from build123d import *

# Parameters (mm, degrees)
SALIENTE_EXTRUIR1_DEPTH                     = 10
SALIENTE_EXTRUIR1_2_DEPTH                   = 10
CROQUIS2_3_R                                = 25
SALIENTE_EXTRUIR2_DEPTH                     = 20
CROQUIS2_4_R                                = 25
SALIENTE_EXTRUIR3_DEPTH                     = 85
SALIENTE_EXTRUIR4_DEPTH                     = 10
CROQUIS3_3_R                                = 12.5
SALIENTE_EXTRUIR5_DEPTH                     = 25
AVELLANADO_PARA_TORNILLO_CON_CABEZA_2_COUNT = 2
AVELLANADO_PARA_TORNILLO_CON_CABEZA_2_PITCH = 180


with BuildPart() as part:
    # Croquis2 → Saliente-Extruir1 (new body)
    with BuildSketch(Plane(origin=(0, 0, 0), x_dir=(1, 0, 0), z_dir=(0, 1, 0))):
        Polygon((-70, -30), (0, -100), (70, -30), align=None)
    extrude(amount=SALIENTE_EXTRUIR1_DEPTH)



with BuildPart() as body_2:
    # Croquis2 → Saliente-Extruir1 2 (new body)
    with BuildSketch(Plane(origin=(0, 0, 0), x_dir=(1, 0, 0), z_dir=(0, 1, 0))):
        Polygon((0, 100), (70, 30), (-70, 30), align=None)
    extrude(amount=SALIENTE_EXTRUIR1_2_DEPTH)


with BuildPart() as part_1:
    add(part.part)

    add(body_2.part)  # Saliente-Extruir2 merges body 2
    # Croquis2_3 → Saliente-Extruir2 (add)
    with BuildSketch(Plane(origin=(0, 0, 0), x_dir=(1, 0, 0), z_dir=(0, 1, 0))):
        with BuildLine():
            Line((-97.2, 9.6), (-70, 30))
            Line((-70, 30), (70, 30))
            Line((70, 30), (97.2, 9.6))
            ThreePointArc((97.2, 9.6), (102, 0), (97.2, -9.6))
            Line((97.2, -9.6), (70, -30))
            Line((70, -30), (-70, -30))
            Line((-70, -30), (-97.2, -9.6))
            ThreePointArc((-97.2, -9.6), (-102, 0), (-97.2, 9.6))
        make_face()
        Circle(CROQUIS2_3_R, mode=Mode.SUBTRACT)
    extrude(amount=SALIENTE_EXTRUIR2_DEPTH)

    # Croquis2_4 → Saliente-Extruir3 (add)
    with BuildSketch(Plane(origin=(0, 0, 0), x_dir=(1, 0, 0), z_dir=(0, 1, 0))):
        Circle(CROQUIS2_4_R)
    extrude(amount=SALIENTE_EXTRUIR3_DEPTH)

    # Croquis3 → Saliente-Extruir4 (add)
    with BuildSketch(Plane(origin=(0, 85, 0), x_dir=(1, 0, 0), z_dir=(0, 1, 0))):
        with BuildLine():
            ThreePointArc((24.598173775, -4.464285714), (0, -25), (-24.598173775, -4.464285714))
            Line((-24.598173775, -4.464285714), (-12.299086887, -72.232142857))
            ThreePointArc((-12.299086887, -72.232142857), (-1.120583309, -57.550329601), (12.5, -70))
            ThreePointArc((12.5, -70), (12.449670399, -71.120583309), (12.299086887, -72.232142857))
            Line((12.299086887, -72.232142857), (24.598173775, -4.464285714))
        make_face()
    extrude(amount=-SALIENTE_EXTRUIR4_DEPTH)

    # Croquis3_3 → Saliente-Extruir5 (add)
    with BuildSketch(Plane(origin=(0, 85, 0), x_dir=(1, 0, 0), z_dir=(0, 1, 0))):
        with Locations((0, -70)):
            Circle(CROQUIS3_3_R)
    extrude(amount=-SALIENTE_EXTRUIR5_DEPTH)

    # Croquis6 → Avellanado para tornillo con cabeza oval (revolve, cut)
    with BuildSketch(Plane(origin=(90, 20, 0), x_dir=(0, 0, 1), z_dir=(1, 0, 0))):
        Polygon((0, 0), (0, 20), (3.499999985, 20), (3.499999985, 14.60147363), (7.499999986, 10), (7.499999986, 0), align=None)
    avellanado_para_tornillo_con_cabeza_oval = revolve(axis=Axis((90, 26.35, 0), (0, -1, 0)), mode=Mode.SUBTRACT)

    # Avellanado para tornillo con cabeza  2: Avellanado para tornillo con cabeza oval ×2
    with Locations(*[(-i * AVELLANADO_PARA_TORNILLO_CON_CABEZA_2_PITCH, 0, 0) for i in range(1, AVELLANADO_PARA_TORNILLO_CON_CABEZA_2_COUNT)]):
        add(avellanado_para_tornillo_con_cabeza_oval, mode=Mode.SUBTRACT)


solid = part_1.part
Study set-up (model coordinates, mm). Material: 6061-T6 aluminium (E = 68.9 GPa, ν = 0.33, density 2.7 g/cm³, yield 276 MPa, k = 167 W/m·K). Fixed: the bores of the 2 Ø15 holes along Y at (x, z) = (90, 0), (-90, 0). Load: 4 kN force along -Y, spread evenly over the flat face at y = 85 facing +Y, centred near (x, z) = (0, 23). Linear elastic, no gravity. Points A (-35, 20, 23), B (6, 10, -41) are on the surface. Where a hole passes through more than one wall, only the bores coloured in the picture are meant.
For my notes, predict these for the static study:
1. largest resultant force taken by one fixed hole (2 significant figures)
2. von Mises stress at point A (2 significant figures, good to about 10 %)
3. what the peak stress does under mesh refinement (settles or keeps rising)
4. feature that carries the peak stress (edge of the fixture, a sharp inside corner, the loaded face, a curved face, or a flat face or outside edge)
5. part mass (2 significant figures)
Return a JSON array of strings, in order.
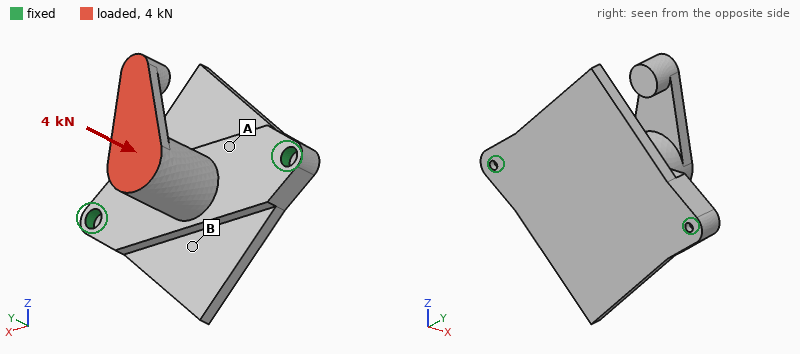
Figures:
["2.5 kN", "12 MPa", "keeps rising", "edge of the fixture", "1.2 kg"]
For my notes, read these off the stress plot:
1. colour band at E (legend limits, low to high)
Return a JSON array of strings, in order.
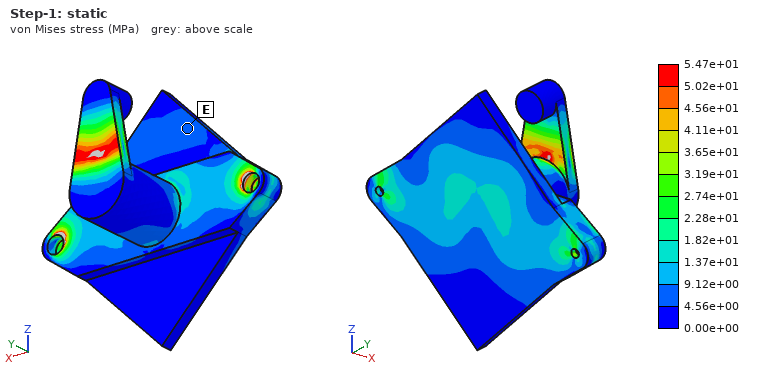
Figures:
["4.56e+00 to 9.12e+00 MPa"]
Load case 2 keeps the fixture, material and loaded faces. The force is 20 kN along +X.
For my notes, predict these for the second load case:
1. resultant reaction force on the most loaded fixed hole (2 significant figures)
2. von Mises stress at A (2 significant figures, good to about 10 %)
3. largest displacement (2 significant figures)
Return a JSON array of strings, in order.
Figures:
["15 kN", "87 MPa", "0.73 mm"]
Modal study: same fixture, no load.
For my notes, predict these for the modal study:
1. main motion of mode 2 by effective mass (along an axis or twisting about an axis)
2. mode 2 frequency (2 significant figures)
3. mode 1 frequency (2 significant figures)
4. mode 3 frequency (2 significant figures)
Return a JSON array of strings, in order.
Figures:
["along Y", "1500 Hz", "910 Hz", "1800 Hz"]
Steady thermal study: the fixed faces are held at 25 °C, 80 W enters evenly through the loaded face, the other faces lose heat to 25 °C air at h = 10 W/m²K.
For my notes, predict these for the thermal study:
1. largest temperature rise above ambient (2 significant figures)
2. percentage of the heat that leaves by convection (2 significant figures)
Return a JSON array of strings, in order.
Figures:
["49 K", "11 %"]
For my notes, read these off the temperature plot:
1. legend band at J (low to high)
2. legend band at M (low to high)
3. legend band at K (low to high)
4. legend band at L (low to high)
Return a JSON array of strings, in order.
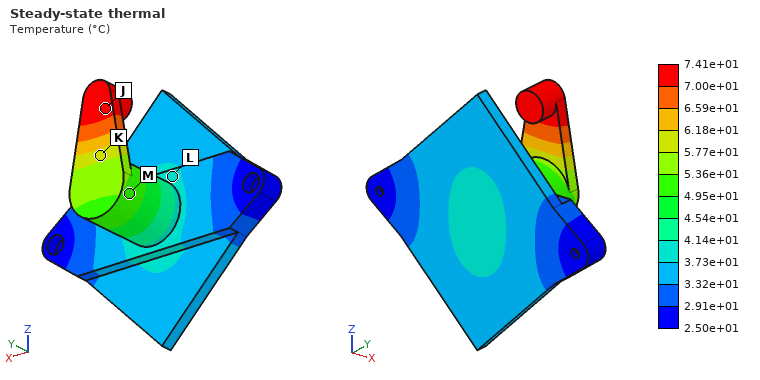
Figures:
["7.00e+01 to 7.41e+01 °C", "4.95e+01 to 5.36e+01 °C", "5.77e+01 to 6.18e+01 °C", "3.73e+01 to 4.14e+01 °C"]
